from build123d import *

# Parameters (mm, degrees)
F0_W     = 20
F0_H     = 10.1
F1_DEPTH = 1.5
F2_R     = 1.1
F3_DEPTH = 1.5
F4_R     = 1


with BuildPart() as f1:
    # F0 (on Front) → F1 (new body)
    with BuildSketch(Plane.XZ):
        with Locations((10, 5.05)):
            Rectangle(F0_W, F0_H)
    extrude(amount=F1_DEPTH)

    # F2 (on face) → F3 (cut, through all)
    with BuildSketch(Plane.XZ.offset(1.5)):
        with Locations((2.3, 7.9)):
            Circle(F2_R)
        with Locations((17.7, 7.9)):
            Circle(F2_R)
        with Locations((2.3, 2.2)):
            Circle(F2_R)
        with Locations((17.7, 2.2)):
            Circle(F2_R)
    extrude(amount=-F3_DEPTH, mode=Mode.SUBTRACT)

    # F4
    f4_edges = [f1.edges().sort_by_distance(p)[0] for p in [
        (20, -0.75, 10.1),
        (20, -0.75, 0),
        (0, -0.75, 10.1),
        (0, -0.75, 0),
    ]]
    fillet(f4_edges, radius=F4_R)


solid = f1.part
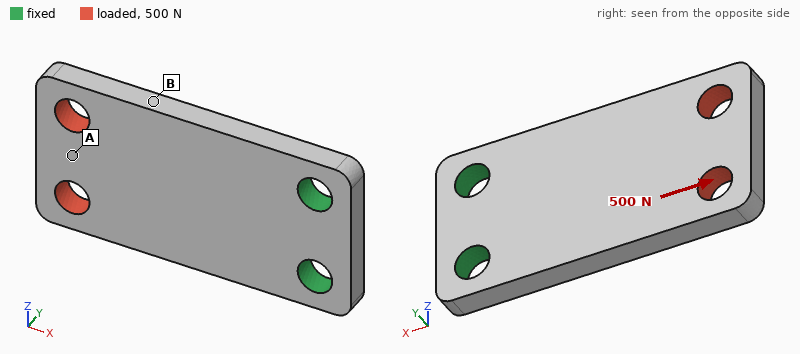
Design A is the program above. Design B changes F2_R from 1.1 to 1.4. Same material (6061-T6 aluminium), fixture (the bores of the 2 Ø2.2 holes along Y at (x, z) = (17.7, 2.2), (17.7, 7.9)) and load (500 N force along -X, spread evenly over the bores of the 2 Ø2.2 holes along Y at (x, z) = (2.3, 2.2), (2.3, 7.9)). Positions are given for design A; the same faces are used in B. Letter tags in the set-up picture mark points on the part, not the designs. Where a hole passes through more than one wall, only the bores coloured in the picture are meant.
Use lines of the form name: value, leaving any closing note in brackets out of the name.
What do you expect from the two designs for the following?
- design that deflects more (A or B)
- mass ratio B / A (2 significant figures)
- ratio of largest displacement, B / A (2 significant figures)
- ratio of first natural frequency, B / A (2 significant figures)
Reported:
design that deflects more: B
mass ratio B / A: 0.95
ratio of largest displacement, B / A: 1.1
ratio of first natural frequency, B / A: 1.1
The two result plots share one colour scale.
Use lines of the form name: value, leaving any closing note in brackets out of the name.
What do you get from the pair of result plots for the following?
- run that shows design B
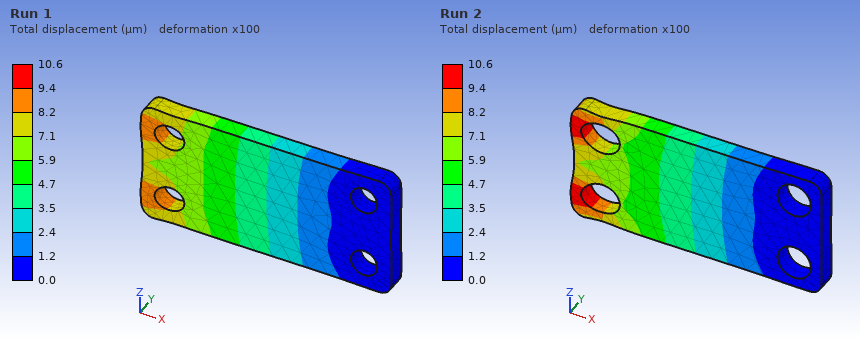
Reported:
run that shows design B: Run 2
